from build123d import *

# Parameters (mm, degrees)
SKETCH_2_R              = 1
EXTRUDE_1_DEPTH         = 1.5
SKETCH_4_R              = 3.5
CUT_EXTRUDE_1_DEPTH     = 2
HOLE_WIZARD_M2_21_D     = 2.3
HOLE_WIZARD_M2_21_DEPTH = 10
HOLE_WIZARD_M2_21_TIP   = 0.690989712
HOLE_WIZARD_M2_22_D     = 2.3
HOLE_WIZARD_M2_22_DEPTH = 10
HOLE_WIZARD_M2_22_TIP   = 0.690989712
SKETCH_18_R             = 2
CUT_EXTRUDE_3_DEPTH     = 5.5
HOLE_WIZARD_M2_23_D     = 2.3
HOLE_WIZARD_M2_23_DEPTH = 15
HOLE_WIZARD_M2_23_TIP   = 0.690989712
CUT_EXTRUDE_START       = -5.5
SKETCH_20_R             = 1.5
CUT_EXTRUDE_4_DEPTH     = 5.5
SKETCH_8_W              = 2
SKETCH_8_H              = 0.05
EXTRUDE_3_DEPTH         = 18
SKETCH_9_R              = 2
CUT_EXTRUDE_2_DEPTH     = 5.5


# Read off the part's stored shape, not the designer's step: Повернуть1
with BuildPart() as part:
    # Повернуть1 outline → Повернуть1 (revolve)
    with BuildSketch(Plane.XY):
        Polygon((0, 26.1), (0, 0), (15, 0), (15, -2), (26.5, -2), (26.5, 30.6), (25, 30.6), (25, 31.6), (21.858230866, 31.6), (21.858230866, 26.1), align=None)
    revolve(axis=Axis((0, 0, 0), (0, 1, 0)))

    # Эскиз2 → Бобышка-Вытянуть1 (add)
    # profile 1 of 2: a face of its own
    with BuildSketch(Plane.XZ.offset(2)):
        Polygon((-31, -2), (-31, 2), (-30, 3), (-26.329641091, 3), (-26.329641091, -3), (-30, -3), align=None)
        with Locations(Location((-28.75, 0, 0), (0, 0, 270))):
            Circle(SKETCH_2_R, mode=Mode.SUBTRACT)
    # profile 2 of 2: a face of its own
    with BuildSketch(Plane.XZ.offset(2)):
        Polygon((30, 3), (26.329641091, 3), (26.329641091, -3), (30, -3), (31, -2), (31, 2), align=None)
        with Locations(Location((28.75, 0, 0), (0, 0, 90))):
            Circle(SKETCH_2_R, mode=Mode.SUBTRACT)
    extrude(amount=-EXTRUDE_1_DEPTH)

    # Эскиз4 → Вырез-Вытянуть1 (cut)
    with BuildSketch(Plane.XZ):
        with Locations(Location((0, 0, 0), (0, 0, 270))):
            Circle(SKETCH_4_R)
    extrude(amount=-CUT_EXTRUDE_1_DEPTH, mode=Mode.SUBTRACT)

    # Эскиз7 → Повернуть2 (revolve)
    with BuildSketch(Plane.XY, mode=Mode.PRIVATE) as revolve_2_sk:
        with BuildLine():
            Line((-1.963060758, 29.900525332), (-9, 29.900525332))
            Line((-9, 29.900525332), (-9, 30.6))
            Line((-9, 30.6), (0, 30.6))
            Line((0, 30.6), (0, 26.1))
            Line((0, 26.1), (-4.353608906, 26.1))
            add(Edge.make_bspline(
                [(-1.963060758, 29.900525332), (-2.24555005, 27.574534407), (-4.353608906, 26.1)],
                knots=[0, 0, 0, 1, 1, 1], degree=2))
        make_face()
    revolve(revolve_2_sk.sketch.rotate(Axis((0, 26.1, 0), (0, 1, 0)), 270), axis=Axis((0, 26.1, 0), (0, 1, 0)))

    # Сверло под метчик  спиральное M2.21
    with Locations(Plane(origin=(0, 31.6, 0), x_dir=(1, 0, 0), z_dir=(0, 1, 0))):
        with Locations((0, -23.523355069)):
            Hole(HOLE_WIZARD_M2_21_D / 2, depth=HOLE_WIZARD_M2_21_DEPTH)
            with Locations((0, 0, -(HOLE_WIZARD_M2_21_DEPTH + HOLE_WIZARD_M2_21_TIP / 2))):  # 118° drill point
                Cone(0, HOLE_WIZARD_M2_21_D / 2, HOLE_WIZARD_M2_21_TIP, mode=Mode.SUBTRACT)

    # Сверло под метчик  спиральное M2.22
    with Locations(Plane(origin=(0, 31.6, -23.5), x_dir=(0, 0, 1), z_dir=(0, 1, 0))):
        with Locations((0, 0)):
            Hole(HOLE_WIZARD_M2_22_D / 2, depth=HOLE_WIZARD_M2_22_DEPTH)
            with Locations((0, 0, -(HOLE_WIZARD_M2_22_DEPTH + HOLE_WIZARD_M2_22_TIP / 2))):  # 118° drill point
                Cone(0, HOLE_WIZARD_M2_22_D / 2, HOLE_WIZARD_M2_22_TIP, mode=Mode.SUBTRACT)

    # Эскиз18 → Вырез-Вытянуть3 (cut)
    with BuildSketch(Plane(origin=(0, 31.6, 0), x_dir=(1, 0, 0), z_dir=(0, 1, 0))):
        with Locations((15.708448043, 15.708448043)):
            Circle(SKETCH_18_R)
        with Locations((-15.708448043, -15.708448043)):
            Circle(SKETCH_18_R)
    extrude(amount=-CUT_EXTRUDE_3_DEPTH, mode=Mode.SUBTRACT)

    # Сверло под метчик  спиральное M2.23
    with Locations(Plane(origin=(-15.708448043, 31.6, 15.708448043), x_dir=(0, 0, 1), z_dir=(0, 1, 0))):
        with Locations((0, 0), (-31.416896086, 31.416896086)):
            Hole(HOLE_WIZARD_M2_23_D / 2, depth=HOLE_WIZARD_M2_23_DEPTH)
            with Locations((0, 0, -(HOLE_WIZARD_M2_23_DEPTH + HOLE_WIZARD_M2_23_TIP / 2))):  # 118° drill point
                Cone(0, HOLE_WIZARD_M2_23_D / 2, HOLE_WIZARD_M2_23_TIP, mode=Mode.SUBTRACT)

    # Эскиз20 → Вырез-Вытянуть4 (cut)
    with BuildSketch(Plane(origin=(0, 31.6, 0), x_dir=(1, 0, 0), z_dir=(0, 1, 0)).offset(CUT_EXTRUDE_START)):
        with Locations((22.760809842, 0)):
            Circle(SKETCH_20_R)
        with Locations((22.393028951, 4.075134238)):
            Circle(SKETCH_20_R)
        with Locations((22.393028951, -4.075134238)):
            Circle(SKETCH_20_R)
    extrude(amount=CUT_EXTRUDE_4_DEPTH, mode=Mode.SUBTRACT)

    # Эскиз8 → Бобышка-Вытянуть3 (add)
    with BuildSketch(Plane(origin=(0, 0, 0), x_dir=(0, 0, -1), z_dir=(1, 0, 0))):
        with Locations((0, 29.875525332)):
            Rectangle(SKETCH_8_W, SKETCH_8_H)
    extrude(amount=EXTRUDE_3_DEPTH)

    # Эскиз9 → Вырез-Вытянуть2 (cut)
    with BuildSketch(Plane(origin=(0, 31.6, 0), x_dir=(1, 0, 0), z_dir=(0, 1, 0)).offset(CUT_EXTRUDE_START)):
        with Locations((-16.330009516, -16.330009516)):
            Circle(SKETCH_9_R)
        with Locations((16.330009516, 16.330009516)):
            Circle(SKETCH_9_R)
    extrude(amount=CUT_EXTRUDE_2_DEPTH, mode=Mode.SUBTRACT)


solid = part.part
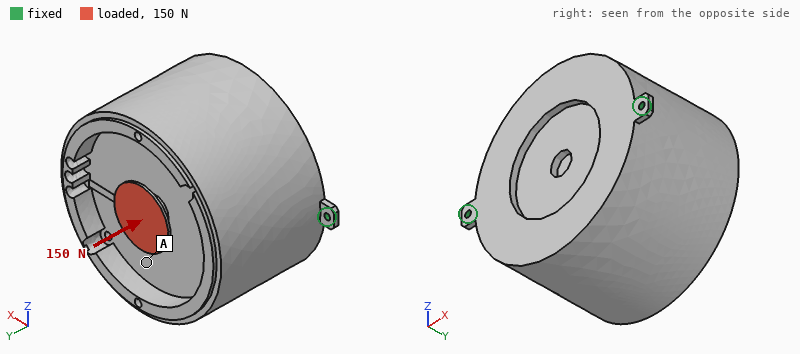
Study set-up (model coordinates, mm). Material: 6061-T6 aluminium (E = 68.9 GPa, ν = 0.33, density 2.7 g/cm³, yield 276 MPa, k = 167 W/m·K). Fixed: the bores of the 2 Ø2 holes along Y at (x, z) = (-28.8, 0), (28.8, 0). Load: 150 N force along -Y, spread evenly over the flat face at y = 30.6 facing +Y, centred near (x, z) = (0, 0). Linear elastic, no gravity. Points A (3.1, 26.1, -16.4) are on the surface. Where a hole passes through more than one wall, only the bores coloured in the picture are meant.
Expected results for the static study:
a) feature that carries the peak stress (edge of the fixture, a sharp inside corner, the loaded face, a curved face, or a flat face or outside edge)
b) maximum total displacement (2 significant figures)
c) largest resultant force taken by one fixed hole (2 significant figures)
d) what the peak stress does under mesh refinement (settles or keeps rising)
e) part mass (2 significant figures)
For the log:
a sharp inside corner
0.19 mm
86 N
keeps rising
170 g
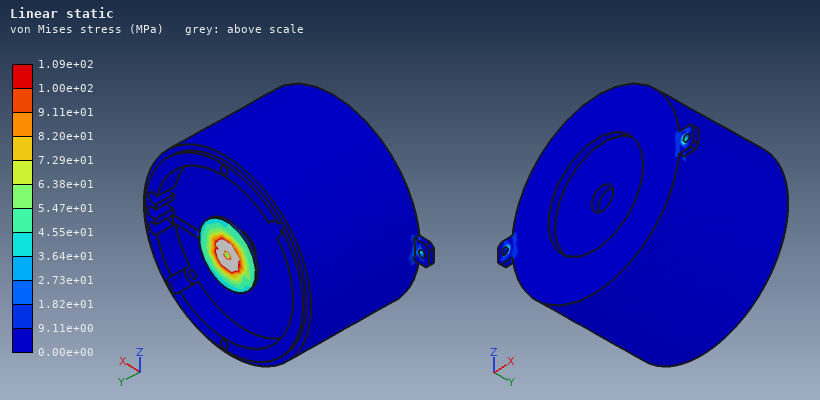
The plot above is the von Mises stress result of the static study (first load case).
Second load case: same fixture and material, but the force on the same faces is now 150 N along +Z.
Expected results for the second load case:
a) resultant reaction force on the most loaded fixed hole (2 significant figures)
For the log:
75 N
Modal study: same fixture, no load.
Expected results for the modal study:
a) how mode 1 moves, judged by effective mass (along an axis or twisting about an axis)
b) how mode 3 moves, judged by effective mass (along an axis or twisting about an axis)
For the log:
along Z
along Y
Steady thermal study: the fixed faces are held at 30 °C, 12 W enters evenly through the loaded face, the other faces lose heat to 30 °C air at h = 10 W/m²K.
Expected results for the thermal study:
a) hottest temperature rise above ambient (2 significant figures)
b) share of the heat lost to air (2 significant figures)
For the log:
52 K
14 %
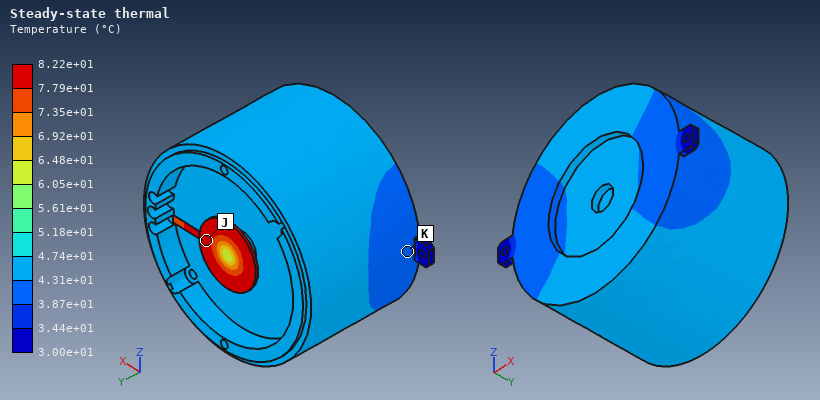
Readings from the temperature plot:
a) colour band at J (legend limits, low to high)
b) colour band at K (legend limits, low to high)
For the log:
7.79e+01 to 8.22e+01 °C
3.87e+01 to 4.31e+01 °C
